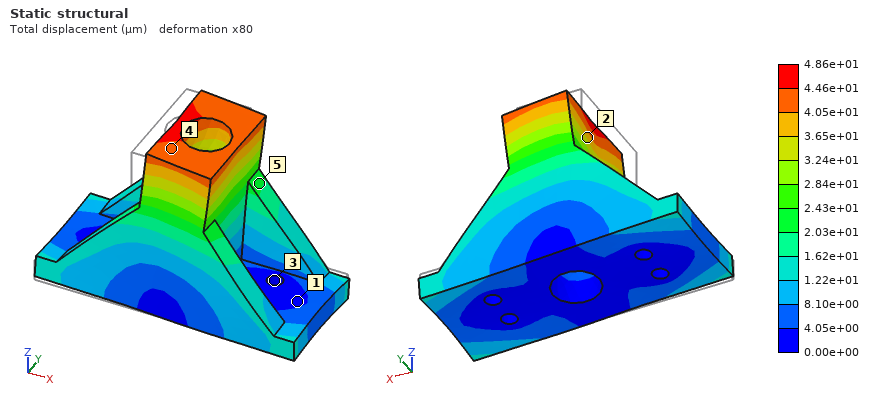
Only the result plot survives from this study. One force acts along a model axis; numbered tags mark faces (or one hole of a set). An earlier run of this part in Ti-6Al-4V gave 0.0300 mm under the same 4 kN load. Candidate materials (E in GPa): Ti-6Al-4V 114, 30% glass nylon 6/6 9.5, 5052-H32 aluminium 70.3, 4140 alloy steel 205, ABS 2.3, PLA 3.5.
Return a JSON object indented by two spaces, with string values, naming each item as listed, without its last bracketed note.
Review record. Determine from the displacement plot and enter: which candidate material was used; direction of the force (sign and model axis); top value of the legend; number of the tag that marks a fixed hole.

{
  "which candidate material was used": "5052-H32 aluminium",
  "direction of the force": "+X",
  "top value of the legend": "4.86e+01 µm",
  "number of the tag that marks a fixed hole": "3"
}
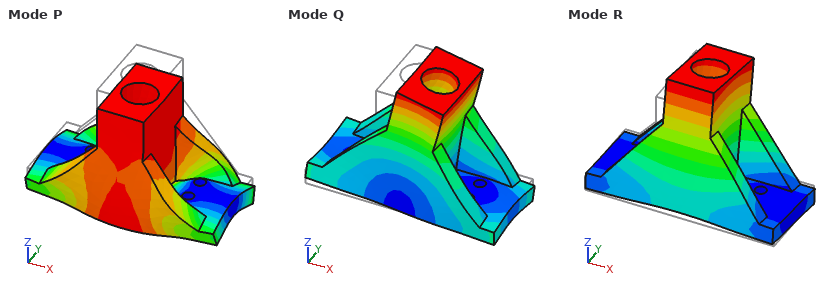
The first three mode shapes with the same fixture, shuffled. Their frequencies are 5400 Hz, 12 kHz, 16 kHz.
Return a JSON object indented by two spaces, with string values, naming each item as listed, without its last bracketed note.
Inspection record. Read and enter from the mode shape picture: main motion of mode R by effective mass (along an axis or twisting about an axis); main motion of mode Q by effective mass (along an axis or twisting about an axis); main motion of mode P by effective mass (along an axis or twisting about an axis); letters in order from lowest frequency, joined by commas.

{
  "main motion of mode R by effective mass": "along Y",
  "main motion of mode Q by effective mass": "along X",
  "main motion of mode P by effective mass": "along Z",
  "letters in order from lowest frequency, joined by commas": "R, Q, P"
}
